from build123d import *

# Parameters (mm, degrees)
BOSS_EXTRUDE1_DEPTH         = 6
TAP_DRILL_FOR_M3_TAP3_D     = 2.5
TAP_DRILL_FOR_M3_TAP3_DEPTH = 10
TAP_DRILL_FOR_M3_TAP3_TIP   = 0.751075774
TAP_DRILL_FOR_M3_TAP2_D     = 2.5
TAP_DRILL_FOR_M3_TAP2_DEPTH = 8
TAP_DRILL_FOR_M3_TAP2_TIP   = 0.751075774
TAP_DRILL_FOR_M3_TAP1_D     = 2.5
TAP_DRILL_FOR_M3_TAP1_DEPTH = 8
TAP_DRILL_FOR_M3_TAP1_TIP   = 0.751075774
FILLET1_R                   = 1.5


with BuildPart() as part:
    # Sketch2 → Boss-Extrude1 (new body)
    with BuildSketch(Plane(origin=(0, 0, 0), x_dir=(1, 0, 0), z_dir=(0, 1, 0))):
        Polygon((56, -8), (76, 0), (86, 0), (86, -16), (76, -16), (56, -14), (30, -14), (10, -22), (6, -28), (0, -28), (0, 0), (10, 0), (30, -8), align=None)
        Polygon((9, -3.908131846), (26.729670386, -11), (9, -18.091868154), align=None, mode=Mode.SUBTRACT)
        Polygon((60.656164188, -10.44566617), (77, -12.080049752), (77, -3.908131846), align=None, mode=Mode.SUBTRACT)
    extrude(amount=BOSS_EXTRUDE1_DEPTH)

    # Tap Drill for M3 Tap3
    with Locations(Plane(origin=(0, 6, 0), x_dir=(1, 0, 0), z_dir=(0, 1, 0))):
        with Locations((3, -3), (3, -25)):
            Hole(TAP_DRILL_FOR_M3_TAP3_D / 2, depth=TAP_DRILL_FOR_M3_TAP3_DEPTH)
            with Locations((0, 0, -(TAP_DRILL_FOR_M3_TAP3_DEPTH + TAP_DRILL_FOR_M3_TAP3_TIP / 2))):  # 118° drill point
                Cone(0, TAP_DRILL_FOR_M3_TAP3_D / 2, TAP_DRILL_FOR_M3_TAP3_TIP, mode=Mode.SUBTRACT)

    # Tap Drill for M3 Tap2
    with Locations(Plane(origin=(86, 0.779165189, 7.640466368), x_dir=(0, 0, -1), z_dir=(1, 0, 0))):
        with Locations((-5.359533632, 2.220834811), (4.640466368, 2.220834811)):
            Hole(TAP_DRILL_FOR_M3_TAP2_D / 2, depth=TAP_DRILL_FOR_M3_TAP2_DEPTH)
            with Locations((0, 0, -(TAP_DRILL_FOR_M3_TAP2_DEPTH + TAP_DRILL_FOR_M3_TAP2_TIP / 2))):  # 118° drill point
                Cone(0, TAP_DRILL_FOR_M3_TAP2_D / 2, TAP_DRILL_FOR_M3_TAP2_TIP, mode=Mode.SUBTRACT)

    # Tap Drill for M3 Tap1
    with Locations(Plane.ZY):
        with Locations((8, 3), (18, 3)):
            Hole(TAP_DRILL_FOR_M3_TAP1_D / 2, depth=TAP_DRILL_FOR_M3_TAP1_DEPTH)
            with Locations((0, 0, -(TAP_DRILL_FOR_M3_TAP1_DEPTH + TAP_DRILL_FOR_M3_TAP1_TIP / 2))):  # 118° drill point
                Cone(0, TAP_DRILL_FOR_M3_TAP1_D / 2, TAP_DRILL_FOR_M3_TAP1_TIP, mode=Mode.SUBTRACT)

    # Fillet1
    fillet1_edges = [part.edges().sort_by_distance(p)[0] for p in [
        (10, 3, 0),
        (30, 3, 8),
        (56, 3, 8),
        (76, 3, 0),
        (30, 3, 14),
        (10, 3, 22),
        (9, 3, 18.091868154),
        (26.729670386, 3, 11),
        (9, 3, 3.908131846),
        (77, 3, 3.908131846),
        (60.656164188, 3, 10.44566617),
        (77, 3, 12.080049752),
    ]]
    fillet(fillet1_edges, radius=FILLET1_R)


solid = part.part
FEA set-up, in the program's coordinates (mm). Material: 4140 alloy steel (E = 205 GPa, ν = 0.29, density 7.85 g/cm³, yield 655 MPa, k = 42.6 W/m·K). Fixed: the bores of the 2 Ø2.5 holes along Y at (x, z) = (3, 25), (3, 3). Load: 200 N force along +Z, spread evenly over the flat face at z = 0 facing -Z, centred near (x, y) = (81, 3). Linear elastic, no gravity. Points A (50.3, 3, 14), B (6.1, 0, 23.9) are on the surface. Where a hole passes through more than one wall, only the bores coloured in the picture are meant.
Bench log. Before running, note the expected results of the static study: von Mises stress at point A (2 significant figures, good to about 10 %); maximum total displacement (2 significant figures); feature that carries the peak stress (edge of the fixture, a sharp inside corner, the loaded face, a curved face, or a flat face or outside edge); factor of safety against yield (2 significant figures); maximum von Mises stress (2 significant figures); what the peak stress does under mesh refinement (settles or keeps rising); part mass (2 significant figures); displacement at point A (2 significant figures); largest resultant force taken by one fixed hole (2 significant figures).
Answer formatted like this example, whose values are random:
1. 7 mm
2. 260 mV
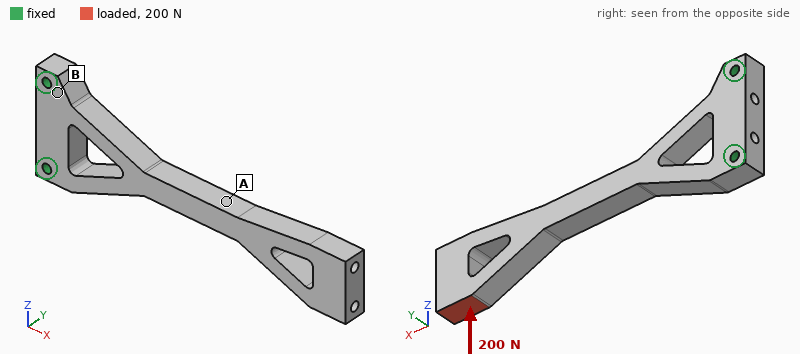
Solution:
1. 170 MPa
2. 0.64 mm
3. a curved face
4. 1.8
5. 360 MPa
6. settles
7. 41 g
8. 0.16 mm
9. 780 N
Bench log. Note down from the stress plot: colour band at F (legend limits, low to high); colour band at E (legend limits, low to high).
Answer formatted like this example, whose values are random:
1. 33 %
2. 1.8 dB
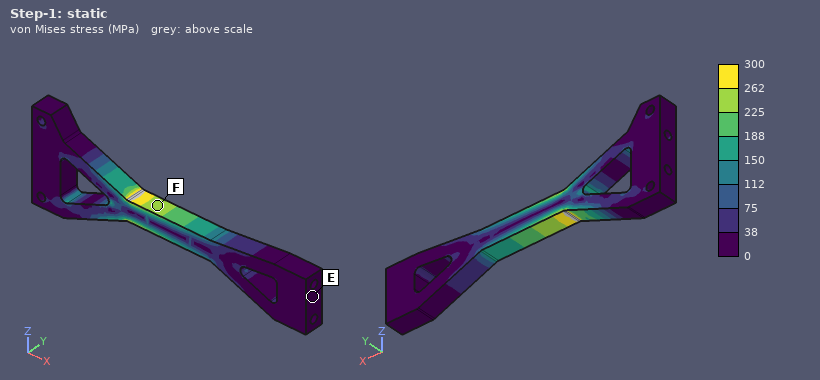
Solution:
1. 225 to 262 MPa
2. 0 to 38 MPa
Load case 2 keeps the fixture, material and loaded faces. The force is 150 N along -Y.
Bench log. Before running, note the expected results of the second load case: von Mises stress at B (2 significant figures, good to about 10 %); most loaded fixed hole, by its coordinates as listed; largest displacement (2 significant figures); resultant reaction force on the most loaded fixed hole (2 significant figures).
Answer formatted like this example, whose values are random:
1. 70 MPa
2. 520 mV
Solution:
1. 120 MPa
2. (3, 3)
3. 1.0 mm
4. 170 N
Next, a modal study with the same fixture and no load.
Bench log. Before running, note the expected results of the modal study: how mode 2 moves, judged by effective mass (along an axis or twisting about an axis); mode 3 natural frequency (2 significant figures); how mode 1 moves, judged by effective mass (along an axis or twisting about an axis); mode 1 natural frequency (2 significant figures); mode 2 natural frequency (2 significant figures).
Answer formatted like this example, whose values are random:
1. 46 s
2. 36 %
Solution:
1. along Z
2. 4100 Hz
3. along Y
4. 610 Hz
5. 930 Hz
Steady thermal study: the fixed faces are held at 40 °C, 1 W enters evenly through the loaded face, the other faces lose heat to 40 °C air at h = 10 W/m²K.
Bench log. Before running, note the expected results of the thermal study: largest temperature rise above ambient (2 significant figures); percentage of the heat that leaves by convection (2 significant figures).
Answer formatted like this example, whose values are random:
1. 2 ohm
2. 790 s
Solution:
1. 29 K
2. 44 %
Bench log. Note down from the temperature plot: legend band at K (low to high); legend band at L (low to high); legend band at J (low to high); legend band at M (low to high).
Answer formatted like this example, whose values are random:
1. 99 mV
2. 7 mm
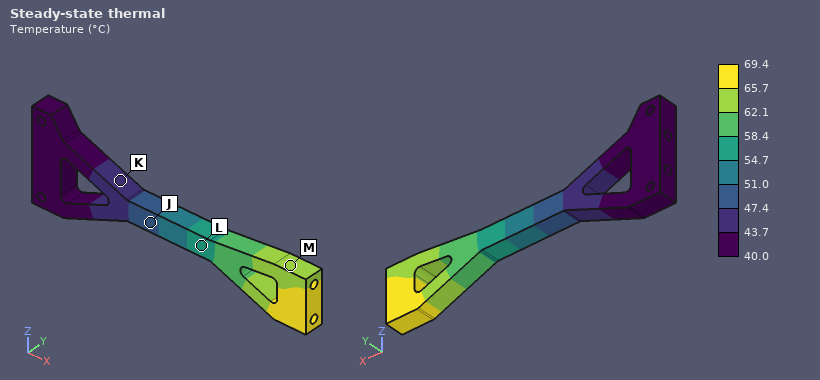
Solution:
1. 43.7 to 47.4 °C
2. 54.7 to 58.4 °C
3. 47.4 to 51.0 °C
4. 62.1 to 65.7 °C
